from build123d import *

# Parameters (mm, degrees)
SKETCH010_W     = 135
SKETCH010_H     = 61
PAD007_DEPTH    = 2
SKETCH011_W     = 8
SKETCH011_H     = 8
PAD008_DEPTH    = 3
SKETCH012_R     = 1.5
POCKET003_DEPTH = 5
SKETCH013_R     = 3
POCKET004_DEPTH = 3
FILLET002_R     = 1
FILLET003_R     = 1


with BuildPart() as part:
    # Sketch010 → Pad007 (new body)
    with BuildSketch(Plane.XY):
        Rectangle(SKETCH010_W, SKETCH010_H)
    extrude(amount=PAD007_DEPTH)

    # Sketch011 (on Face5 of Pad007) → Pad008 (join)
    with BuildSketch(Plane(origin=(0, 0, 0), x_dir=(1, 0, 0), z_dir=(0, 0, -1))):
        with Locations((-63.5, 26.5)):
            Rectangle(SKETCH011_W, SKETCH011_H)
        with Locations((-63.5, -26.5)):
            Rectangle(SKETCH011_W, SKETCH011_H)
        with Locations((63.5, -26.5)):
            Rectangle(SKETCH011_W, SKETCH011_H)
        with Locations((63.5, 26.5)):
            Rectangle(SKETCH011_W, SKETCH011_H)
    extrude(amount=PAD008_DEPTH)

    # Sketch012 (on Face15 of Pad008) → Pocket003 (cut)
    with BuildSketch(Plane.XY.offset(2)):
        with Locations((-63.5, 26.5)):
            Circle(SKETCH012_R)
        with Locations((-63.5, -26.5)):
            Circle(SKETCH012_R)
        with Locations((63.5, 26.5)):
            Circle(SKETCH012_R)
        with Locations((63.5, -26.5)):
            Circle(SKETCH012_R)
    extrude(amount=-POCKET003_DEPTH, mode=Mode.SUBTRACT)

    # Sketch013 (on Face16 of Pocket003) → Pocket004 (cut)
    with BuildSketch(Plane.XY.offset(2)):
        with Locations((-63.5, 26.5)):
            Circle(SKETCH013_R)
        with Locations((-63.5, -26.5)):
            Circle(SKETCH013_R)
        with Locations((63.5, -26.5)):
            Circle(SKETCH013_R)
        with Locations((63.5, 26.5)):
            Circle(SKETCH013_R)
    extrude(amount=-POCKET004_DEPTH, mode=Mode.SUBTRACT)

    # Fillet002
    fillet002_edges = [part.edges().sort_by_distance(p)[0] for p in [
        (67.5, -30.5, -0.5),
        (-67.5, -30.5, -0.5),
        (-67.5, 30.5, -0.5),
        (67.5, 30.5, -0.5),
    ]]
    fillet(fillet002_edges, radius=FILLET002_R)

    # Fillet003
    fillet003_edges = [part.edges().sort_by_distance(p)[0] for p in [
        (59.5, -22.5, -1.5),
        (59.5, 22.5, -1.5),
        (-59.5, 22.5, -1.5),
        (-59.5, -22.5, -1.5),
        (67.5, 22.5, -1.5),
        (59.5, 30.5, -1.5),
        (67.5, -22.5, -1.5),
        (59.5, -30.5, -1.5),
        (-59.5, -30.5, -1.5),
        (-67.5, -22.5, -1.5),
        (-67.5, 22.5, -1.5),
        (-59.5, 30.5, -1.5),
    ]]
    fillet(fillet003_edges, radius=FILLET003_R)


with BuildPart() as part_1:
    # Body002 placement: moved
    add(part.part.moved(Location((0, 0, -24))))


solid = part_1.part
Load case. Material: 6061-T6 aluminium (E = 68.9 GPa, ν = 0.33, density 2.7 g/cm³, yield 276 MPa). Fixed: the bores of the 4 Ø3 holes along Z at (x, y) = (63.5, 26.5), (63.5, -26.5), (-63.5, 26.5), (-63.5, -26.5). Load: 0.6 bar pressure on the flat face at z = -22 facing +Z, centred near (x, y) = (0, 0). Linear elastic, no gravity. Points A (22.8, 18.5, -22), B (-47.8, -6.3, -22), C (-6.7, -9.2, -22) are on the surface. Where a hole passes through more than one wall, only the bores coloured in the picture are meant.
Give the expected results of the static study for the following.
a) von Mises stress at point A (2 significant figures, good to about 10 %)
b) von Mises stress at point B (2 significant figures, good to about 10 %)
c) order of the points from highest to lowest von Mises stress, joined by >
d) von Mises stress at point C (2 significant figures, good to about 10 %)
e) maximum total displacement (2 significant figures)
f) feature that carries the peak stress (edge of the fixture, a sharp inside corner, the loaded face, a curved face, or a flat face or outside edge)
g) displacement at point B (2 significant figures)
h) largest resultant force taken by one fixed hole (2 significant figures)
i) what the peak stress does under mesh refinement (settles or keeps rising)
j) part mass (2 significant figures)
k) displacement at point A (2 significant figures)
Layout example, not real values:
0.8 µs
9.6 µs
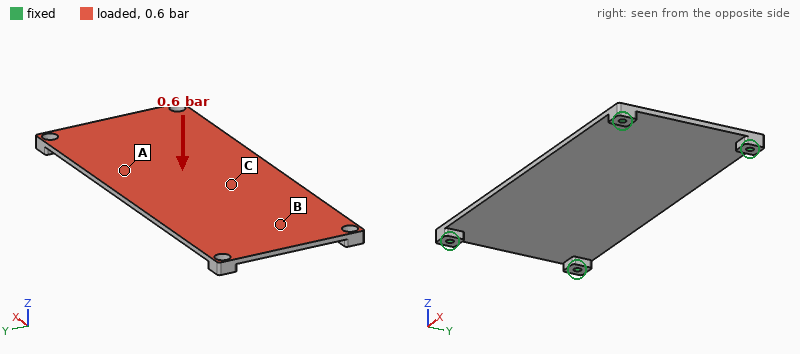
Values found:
48 MPa
32 MPa
C > A > B
63 MPa
1.1 mm
a sharp inside corner
0.27 mm
380 N
keeps rising
45 g
0.79 mm
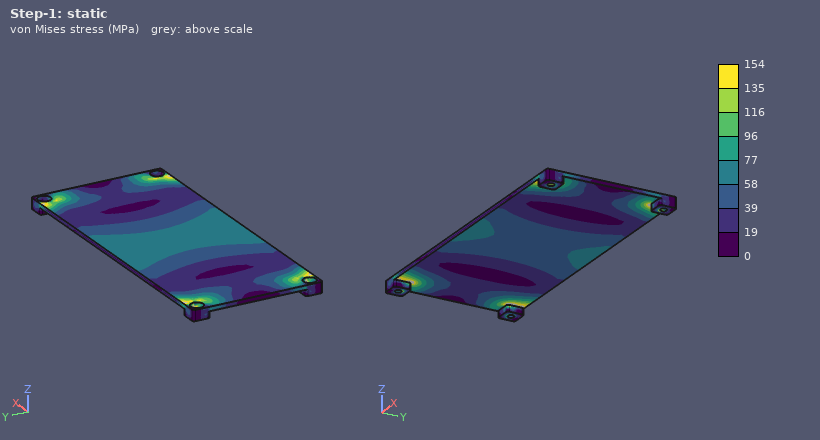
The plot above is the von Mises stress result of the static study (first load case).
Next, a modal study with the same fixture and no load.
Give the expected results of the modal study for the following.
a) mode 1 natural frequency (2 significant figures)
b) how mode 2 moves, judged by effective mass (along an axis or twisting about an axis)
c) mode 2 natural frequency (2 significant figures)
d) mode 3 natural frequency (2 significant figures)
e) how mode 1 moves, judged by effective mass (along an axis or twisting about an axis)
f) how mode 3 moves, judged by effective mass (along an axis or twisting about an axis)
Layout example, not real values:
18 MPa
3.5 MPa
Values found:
600 Hz
twisting about X
1100 Hz
1600 Hz
along Z
twisting about Y
